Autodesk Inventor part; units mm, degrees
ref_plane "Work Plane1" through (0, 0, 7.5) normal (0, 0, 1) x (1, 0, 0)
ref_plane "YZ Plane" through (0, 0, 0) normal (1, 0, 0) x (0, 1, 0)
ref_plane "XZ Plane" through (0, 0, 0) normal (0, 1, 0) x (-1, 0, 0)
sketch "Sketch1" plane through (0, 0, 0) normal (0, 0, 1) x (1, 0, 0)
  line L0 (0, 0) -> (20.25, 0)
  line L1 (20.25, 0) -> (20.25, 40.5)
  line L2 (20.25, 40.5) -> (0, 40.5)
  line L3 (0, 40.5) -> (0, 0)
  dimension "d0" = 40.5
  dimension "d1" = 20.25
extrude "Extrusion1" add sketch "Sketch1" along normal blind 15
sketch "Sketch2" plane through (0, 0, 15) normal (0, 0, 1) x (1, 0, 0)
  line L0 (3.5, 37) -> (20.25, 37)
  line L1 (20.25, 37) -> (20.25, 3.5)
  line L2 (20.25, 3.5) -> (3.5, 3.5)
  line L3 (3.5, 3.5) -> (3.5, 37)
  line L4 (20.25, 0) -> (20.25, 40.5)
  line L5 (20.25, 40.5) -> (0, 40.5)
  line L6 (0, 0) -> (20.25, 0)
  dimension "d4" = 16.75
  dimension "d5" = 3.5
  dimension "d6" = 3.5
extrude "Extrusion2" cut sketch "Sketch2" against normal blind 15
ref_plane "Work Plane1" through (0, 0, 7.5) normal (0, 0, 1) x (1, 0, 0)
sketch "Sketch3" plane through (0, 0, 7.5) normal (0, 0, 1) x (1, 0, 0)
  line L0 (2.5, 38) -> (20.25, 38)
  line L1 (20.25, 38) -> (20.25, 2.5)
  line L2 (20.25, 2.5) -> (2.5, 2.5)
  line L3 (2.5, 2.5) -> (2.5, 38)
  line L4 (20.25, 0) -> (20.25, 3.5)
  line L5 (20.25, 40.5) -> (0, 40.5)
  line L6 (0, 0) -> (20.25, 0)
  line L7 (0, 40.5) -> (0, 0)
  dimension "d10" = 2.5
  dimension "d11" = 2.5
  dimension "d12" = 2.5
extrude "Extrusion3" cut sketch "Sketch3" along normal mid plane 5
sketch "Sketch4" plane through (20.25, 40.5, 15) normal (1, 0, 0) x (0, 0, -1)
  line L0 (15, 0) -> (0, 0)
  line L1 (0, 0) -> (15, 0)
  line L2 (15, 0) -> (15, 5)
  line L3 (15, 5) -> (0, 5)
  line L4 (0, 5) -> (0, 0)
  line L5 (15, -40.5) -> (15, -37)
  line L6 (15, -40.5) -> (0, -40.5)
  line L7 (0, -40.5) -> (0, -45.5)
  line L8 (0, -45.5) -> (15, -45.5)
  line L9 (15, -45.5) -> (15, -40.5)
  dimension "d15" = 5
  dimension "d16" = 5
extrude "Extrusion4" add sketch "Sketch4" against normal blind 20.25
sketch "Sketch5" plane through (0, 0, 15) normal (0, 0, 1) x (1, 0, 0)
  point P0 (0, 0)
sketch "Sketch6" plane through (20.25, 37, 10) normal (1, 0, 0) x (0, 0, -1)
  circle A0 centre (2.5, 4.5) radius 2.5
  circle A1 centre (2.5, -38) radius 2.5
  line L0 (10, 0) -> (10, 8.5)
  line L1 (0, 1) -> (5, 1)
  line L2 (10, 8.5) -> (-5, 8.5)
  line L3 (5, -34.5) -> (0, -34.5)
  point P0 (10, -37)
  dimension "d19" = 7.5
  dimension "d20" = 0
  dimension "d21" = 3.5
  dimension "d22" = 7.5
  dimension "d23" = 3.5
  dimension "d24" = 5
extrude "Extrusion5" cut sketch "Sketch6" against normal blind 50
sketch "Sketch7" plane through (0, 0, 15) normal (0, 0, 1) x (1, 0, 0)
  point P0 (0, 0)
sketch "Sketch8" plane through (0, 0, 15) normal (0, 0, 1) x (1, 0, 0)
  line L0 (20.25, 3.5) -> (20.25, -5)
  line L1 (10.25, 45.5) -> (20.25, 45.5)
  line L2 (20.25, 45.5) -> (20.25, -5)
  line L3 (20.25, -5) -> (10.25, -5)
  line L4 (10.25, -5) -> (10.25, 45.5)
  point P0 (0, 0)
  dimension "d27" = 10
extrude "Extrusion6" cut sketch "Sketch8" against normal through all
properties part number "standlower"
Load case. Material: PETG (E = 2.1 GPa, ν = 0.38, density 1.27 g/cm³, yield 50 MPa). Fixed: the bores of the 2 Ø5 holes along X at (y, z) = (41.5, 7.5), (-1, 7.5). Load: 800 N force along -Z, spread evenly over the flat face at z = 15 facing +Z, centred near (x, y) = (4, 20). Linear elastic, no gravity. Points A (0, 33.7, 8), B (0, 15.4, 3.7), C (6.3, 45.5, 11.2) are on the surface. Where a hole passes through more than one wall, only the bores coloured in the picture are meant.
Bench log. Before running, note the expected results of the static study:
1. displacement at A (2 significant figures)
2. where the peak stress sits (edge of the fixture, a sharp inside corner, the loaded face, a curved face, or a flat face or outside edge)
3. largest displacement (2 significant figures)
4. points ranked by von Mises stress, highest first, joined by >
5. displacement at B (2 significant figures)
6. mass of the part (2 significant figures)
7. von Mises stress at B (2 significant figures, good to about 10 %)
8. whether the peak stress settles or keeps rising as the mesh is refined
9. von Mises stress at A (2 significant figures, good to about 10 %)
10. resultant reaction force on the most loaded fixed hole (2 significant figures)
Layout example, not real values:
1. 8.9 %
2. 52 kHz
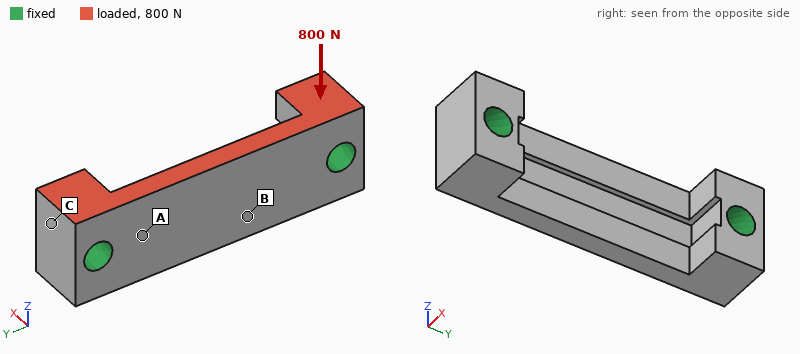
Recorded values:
1. 0.051 mm
2. edge of the fixture
3. 0.15 mm
4. A > B > C
5. 0.11 mm
6. 4.7 g
7. 3.4 MPa
8. keeps rising
9. 6.2 MPa
10. 400 N
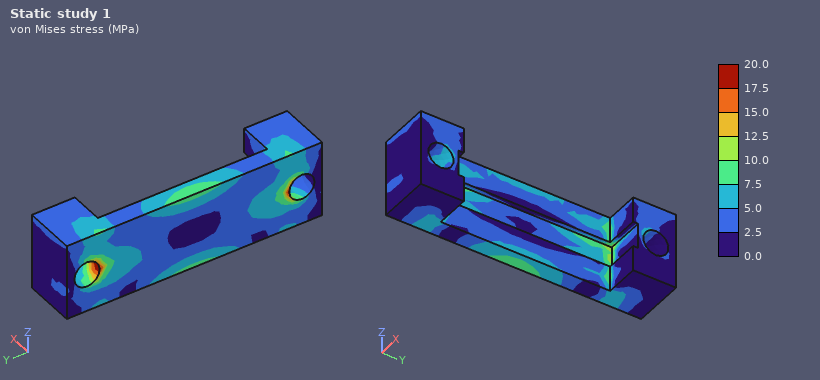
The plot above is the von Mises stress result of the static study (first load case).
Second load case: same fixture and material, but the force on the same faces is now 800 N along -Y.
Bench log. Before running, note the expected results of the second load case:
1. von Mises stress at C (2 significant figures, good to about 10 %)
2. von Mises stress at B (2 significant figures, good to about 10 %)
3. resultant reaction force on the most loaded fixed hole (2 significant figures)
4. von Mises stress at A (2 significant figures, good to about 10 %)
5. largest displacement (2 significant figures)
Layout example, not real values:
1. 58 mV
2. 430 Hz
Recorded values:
1. 7.5 MPa
2. 2.0 MPa
3. 410 N
4. 5.8 MPa
5. 64 µm
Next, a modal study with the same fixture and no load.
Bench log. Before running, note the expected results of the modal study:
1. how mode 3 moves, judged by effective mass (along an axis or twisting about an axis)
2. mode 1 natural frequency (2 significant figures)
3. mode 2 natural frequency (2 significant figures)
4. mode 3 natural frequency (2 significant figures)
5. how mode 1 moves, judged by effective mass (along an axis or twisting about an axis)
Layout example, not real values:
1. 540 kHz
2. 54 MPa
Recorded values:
1. along Z
2. 3100 Hz
3. 4800 Hz
4. 6500 Hz
5. along X
